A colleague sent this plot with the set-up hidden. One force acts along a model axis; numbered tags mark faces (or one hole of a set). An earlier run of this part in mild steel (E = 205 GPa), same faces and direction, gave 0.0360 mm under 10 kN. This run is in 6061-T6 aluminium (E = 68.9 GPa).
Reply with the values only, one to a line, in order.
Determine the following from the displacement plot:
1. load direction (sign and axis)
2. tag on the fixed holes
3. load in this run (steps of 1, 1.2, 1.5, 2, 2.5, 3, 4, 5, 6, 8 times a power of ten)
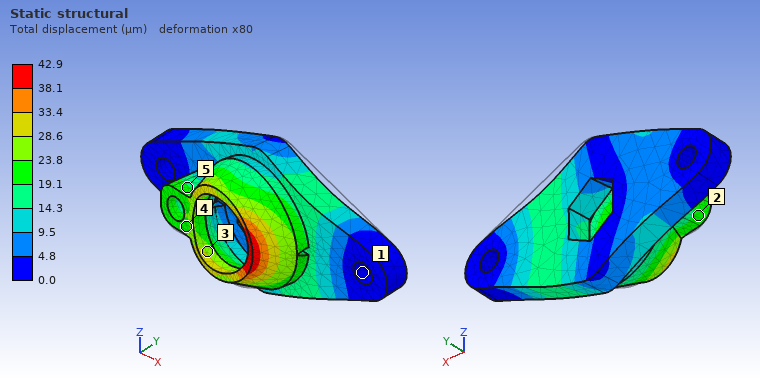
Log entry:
-X
1
4 kN
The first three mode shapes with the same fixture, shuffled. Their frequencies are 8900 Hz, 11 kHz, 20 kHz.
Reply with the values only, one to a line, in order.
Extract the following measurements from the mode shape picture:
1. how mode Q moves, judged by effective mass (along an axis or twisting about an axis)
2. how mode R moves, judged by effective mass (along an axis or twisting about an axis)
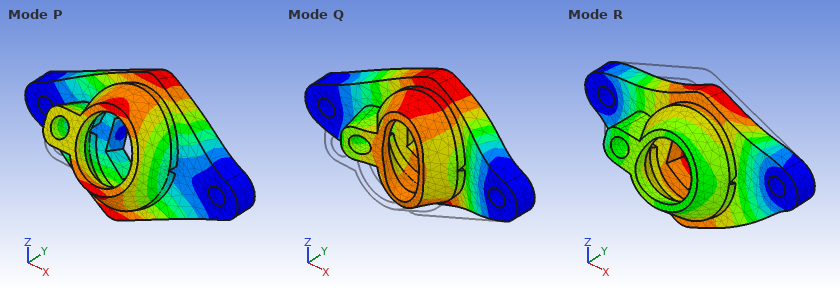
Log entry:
along Y
along Z
